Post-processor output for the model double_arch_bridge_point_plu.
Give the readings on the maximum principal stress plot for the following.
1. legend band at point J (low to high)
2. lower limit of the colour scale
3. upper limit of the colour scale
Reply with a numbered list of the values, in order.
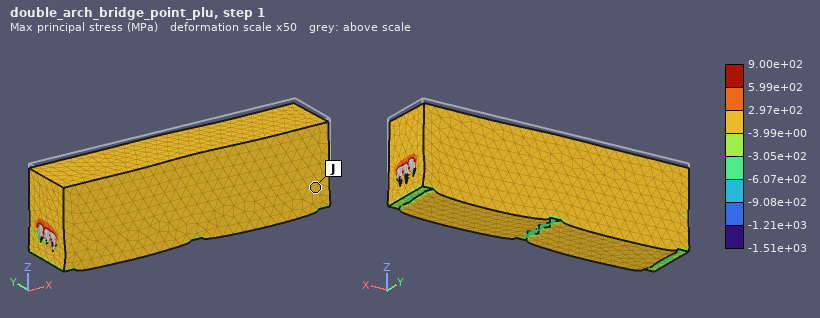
1. -3.99e+00 to 2.97e+02 MPa
2. -1.51e+03 MPa
3. 9.00e+02 MPa
